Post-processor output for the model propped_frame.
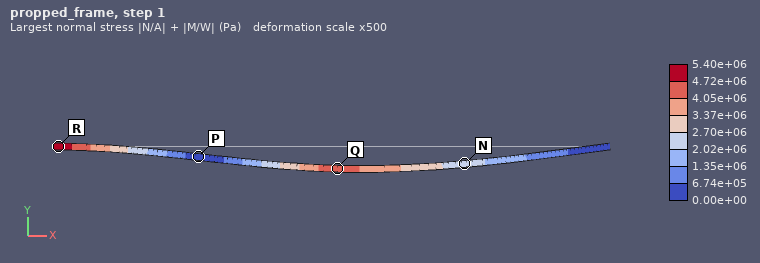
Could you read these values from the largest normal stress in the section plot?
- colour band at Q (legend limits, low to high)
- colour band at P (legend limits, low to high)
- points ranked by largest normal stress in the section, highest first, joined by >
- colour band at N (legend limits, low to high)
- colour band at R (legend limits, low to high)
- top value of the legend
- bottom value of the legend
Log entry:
4.05e+06 to 4.72e+06 Pa
0.00e+00 to 6.74e+05 Pa
R > Q > N > P
2.02e+06 to 2.70e+06 Pa
4.72e+06 to 5.40e+06 Pa
5.40e+06 Pa
0.00e+00 Pa
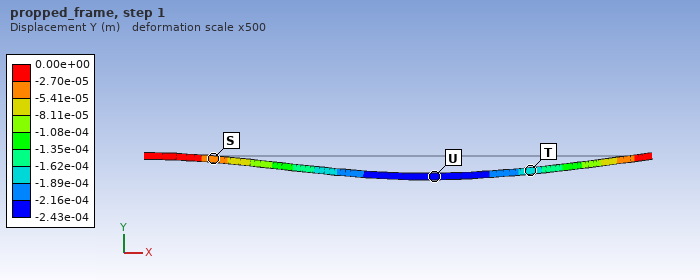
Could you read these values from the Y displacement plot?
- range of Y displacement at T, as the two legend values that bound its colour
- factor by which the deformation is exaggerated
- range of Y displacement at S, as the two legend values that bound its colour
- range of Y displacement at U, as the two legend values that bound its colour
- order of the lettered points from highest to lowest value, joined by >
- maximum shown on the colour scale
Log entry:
-1.89e-04 to -1.62e-04 m
500
-5.41e-05 to -2.70e-05 m
-2.43e-04 to -2.16e-04 m
S > T > U
0.00e+00 m
